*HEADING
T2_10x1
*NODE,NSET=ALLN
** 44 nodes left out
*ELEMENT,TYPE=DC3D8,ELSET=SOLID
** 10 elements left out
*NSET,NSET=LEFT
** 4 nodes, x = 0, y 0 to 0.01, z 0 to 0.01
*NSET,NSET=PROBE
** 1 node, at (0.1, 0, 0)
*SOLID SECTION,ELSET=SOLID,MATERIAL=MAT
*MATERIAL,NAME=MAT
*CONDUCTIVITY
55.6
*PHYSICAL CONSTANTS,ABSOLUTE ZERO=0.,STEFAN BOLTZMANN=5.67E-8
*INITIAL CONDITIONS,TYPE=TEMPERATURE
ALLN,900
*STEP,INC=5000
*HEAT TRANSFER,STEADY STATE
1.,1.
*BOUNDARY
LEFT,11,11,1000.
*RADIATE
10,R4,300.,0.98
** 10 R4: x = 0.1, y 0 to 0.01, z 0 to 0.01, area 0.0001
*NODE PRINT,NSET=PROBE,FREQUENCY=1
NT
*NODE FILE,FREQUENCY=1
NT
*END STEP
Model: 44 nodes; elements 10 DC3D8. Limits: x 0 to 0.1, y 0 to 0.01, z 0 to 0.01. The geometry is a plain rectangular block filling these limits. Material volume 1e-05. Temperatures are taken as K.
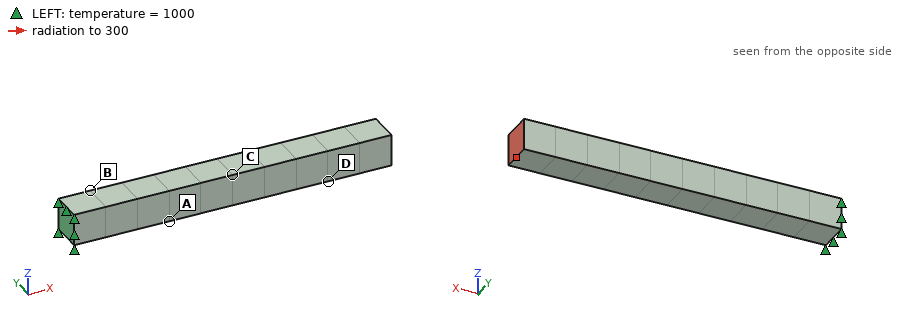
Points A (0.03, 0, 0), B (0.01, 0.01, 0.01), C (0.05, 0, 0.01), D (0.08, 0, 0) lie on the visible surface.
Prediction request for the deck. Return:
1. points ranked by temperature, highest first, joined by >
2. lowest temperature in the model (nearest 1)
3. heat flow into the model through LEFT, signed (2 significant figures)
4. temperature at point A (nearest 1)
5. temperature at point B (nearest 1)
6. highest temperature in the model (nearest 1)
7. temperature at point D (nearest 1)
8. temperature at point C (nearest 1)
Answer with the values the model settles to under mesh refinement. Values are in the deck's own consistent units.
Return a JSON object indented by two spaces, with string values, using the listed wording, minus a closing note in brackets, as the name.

{
  "points ranked by temperature, highest first, joined by >": "B > A > C > D",
  "lowest temperature in the model": "927 K",
  "heat flow into the model through LEFT, signed": "4.1",
  "temperature at point A": "978 K",
  "temperature at point B": "993 K",
  "highest temperature in the model": "1000 K",
  "temperature at point D": "942 K",
  "temperature at point C": "964 K"
}
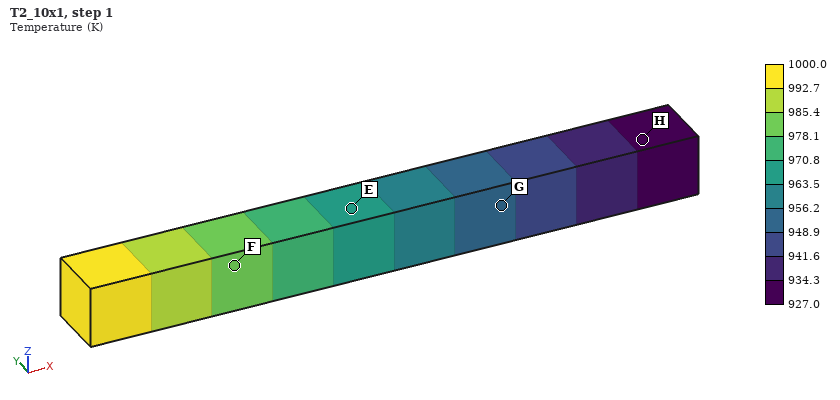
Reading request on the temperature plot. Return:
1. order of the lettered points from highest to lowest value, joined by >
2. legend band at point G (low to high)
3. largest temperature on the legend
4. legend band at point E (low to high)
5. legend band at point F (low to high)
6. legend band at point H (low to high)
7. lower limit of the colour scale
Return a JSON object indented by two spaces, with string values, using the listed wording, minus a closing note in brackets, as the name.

{
  "order of the lettered points from highest to lowest value, joined by >": "F > E > G > H",
  "legend band at point G": "948.9 to 956.2 K",
  "largest temperature on the legend": "1000.0 K",
  "legend band at point E": "963.5 to 970.8 K",
  "legend band at point F": "978.1 to 985.4 K",
  "legend band at point H": "927.0 to 934.3 K",
  "lower limit of the colour scale": "927.0 K"
}
